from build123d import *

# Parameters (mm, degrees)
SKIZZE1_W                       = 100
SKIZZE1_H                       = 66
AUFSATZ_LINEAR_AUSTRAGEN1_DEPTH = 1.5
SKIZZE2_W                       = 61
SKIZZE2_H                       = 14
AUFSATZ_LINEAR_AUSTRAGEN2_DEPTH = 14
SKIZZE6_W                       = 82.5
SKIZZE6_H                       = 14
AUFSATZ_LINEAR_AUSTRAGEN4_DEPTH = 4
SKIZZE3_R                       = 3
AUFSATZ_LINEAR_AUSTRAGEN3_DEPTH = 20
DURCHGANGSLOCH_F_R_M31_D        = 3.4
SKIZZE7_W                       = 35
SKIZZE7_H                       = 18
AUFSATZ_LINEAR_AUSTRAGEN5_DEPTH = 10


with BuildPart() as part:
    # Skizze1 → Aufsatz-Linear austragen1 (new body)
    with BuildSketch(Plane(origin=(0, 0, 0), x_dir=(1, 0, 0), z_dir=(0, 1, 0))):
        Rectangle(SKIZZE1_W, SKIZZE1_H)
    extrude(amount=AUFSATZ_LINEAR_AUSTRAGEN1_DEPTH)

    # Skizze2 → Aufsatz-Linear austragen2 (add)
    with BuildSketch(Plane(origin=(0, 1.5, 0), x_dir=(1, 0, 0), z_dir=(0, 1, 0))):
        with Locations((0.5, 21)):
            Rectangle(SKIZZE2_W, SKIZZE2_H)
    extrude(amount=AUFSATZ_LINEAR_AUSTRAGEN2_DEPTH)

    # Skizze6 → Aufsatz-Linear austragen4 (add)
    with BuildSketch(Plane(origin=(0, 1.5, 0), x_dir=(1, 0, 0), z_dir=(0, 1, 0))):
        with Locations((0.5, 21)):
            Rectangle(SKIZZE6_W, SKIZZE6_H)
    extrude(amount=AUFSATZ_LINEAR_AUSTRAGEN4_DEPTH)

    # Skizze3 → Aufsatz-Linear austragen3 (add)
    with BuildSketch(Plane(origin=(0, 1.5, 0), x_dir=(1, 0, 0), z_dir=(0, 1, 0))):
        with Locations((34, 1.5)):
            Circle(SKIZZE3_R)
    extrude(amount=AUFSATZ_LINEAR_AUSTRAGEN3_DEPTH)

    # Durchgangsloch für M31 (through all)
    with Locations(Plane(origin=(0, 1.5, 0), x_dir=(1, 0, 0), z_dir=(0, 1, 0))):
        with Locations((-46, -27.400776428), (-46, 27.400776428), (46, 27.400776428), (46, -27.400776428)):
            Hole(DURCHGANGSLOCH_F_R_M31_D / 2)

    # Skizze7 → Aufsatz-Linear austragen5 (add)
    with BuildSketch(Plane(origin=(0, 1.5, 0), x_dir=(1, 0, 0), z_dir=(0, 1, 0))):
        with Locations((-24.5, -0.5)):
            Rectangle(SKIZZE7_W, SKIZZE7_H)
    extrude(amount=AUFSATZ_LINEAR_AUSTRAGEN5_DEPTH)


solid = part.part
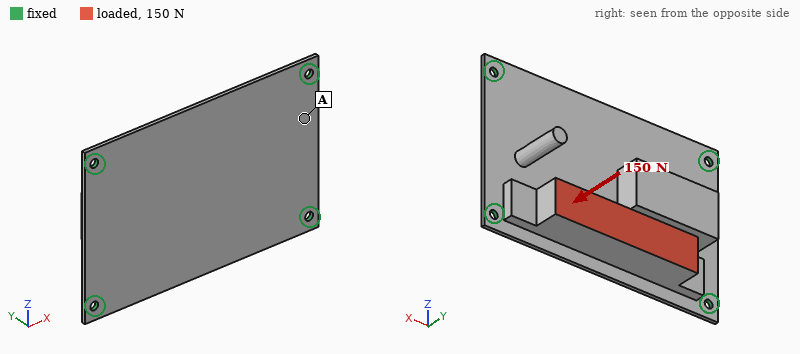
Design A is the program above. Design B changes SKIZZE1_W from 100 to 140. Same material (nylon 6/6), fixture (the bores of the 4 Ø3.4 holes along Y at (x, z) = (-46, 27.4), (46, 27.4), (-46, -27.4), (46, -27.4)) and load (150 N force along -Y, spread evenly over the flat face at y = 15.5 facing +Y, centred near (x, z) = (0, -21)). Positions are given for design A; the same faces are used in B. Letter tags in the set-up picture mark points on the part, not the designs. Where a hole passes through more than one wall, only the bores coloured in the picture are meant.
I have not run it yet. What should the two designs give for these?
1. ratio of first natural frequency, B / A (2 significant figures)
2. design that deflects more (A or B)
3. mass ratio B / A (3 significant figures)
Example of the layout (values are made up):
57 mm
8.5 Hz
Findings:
1.1
A
1.13
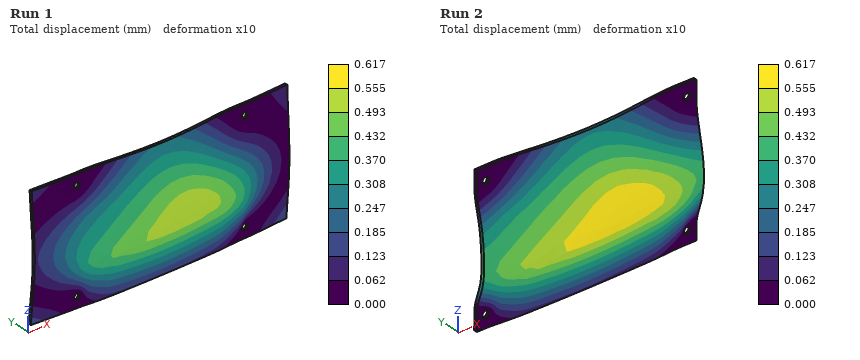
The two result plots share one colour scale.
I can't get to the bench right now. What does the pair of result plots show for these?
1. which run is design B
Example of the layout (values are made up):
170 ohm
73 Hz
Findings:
Run 1
